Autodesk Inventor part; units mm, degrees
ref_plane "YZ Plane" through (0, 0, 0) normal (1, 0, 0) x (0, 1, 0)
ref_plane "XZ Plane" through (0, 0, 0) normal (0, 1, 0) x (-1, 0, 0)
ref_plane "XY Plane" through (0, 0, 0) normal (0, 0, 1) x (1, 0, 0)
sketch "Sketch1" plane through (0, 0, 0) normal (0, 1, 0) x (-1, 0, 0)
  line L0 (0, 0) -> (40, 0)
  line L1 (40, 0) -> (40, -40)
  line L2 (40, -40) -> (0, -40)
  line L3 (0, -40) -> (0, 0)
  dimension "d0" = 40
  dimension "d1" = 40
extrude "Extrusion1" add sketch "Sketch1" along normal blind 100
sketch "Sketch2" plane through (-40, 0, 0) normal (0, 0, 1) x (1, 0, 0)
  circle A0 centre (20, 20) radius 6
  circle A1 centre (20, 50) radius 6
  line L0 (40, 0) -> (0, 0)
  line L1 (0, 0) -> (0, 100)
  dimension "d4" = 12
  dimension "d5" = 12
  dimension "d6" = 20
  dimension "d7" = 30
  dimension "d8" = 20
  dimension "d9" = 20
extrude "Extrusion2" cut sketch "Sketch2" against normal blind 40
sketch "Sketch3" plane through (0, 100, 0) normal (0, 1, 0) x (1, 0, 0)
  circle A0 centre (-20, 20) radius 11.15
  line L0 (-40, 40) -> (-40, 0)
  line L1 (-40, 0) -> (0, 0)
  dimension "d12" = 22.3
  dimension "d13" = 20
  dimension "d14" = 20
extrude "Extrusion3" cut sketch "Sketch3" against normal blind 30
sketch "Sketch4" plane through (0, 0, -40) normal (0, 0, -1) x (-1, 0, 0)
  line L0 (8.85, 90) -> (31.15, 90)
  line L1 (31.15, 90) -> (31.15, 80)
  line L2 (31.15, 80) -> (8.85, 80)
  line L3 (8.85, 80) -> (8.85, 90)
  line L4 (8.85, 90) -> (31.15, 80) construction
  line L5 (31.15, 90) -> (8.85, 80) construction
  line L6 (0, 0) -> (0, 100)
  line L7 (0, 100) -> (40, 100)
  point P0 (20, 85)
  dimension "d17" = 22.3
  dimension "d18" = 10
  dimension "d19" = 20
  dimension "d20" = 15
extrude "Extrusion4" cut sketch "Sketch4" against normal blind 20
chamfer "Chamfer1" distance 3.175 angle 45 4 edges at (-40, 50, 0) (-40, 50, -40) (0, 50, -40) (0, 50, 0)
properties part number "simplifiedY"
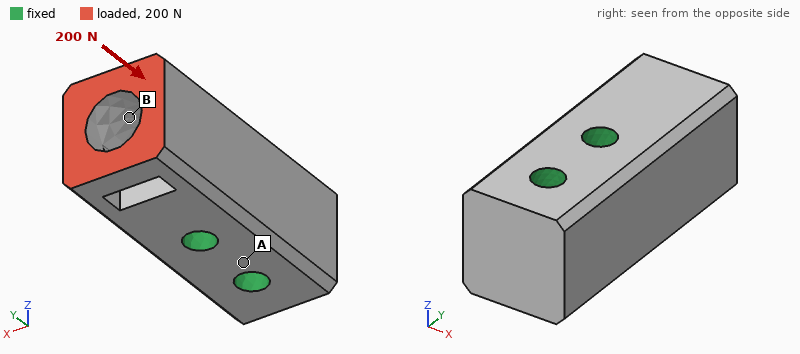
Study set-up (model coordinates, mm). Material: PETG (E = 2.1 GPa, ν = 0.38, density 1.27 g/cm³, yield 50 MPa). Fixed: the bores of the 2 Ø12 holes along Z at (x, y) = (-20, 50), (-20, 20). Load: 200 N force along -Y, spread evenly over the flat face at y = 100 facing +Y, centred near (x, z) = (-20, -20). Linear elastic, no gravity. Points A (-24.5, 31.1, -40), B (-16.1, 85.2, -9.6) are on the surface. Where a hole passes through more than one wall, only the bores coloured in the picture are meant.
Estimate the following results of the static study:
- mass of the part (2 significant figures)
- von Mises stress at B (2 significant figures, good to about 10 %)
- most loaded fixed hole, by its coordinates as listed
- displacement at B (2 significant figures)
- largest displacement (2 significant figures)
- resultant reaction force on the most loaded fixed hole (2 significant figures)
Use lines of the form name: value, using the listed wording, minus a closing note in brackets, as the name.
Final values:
mass of the part: 170 g
von Mises stress at B: 0.21 MPa
most loaded fixed hole, by its coordinates as listed: (-20, 50)
displacement at B: 2.9 µm
largest displacement: 12 µm
resultant reaction force on the most loaded fixed hole: 170 N
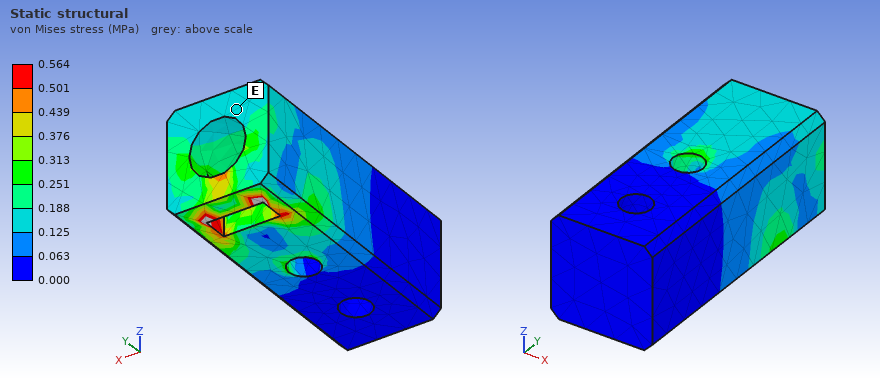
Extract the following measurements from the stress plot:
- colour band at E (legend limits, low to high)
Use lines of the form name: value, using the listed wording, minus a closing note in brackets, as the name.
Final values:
colour band at E: 0.125 to 0.188 MPa
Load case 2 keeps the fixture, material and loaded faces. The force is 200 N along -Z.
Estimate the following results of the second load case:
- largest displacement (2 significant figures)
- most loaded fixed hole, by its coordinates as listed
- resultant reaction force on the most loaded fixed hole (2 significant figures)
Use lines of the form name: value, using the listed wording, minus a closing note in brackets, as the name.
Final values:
largest displacement: 50 µm
most loaded fixed hole, by its coordinates as listed: (-20, 50)
resultant reaction force on the most loaded fixed hole: 230 N
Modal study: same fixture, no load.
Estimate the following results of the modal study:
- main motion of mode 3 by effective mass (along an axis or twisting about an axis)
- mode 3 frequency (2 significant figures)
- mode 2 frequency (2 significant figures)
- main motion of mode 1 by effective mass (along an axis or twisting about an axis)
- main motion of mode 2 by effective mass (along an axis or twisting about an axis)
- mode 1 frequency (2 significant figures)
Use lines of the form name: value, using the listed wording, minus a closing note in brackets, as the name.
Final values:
main motion of mode 3 by effective mass: twisting about Y
mode 3 frequency: 3600 Hz
mode 2 frequency: 2500 Hz
main motion of mode 1 by effective mass: along X
main motion of mode 2 by effective mass: along Z
mode 1 frequency: 2000 Hz
